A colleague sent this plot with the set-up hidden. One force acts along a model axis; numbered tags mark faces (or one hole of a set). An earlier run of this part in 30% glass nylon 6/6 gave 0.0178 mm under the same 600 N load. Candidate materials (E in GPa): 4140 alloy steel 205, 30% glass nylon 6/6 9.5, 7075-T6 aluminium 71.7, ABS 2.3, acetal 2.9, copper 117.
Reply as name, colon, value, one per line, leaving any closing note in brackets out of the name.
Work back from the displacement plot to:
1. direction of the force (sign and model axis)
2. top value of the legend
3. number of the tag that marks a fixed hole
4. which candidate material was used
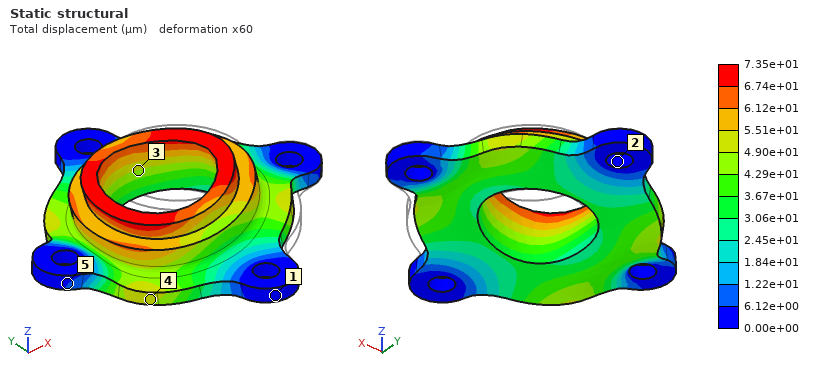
direction of the force: -X
top value of the legend: 7.35e+01 µm
number of the tag that marks a fixed hole: 2
which candidate material was used: ABS
